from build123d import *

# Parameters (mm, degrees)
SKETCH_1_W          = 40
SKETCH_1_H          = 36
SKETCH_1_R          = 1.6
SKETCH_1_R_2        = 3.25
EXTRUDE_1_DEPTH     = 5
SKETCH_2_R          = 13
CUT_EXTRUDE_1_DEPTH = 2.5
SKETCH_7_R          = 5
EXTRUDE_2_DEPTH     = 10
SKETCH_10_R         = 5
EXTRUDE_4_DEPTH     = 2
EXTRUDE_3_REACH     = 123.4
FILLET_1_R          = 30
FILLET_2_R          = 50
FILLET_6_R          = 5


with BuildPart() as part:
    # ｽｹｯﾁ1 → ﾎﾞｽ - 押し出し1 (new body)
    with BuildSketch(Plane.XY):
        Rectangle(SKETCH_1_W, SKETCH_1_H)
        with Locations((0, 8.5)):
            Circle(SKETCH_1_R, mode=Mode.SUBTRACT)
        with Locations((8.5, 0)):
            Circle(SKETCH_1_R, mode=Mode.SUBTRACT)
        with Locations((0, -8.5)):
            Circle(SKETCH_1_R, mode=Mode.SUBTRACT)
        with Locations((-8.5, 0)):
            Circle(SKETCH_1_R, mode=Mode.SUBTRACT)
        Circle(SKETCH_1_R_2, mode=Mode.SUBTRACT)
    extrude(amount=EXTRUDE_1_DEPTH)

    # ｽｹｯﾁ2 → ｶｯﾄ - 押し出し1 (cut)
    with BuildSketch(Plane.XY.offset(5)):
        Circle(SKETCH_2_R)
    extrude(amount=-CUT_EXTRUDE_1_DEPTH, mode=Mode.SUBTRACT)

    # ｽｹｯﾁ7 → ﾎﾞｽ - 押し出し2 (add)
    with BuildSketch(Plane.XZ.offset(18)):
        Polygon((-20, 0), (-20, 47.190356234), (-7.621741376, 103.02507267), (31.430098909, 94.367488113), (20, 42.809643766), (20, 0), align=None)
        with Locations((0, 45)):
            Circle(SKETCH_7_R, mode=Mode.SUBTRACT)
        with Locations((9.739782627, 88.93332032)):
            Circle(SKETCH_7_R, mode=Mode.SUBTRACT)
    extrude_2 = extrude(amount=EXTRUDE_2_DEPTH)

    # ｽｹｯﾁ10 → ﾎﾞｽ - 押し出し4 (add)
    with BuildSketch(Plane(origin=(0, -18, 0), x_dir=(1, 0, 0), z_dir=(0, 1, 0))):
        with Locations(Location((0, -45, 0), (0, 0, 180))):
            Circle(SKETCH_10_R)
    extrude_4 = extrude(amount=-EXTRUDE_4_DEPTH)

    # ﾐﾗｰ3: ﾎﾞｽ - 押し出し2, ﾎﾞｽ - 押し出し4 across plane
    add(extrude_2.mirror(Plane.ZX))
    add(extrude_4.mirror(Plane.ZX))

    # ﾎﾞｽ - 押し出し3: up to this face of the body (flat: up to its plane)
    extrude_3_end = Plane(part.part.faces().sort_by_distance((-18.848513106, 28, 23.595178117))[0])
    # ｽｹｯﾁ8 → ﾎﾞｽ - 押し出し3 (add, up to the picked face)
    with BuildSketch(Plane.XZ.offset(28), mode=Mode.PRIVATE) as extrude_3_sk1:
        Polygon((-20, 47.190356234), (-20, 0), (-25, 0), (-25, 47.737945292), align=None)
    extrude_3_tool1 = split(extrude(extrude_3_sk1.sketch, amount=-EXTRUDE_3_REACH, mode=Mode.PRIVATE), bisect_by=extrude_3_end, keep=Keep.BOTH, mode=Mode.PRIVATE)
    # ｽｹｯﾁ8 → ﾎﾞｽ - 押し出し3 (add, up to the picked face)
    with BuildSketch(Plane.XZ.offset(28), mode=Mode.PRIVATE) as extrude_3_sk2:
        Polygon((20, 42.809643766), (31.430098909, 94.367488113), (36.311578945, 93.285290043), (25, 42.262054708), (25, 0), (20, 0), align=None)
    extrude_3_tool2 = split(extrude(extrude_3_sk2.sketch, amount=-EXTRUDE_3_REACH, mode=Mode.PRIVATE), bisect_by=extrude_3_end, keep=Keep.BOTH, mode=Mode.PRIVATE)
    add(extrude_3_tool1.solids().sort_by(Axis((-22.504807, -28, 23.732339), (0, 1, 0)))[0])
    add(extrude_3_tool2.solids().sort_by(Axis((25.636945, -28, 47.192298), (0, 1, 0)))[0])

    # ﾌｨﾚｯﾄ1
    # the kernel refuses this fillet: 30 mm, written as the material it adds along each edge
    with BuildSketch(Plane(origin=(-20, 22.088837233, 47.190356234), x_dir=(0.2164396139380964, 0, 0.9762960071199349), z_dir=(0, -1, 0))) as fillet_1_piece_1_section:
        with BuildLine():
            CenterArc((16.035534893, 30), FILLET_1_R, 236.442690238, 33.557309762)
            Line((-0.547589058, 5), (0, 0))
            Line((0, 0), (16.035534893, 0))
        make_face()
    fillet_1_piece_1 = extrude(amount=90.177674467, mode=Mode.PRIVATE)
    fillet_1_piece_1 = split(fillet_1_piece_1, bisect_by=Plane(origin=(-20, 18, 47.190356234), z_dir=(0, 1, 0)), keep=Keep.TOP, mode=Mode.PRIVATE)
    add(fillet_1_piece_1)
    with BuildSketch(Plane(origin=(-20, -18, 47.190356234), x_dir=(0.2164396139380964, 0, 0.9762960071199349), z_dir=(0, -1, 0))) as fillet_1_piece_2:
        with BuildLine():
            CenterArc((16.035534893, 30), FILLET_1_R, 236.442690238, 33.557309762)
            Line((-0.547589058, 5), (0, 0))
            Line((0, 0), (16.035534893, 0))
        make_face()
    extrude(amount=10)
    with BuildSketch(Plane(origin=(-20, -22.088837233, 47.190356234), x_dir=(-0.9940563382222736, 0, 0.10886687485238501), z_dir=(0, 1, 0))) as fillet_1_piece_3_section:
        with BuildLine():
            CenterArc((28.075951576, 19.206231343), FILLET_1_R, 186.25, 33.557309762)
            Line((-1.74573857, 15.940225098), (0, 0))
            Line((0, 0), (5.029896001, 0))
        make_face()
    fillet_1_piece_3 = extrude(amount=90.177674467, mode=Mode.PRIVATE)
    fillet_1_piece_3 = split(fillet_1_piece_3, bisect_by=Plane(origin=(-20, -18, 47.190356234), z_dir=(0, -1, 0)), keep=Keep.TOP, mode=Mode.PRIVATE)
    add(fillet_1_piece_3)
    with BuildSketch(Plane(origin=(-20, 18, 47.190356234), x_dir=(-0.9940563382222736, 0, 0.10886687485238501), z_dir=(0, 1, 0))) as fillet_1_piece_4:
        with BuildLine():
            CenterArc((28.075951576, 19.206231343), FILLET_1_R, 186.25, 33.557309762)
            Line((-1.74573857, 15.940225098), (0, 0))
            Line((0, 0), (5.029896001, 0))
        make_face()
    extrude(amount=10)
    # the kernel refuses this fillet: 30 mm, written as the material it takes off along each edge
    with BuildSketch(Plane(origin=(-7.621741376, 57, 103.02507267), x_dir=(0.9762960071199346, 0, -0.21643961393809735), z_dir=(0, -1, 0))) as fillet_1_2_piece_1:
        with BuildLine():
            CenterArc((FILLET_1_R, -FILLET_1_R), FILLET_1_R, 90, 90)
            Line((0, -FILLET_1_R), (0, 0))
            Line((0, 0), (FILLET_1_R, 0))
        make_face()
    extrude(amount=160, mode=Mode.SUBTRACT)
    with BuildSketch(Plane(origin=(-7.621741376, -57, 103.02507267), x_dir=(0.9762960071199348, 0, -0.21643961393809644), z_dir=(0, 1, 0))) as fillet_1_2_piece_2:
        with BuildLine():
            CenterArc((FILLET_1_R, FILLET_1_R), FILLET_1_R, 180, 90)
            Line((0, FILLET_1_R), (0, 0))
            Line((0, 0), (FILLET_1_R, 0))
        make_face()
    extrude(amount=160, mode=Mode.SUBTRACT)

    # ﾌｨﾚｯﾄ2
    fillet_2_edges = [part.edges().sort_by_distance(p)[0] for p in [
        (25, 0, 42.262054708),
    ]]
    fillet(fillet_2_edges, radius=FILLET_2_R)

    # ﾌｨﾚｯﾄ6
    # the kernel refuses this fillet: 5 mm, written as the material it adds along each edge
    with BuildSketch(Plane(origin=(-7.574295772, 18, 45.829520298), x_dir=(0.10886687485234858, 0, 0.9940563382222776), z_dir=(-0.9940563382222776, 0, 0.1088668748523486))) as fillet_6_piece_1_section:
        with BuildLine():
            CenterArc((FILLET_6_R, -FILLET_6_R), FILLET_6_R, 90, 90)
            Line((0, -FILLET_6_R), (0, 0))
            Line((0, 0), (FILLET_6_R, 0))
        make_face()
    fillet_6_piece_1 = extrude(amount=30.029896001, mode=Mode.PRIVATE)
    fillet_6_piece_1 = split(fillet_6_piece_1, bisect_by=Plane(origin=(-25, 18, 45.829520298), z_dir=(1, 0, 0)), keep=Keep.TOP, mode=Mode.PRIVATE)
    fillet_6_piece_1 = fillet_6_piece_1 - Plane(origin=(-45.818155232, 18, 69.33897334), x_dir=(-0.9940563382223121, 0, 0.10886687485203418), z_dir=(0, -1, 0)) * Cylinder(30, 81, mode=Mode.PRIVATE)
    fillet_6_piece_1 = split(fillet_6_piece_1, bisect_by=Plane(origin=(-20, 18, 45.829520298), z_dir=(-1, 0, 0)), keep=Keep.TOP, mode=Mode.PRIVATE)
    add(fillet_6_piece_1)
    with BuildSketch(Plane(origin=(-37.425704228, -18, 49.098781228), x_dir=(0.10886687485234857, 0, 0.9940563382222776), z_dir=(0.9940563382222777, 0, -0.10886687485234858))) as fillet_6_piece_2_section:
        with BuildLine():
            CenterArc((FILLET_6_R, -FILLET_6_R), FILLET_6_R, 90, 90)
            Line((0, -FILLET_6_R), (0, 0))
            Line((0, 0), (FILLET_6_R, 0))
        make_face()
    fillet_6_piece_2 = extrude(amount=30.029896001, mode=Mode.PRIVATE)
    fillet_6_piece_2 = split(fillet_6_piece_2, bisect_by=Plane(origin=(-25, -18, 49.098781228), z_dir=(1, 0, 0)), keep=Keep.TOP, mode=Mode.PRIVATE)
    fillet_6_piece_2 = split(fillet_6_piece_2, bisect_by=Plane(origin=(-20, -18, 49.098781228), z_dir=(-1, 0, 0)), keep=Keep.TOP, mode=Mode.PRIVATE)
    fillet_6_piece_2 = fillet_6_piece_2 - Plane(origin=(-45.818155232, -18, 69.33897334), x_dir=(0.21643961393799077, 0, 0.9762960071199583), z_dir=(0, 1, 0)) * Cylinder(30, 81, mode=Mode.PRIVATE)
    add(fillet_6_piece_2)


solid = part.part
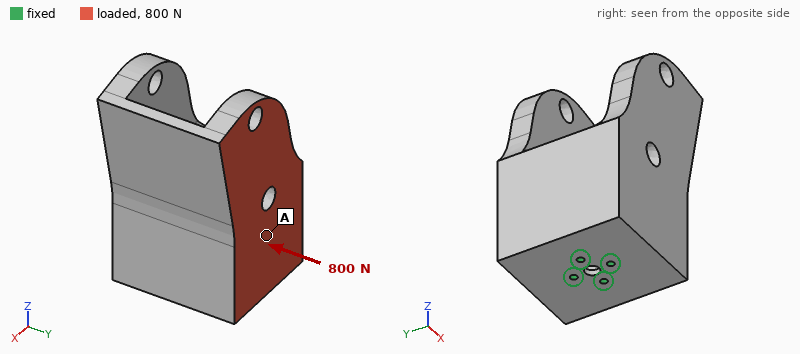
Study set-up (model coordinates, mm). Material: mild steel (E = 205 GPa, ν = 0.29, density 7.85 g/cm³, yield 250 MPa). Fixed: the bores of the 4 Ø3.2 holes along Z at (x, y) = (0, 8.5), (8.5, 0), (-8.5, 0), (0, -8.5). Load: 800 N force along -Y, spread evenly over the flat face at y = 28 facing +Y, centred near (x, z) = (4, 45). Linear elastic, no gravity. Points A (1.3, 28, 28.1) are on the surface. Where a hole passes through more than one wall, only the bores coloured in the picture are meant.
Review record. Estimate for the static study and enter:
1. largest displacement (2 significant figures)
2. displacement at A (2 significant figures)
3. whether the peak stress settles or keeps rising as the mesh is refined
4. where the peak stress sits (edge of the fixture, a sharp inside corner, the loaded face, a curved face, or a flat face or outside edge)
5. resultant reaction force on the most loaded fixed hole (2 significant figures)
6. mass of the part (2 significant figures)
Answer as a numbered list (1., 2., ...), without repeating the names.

1. 0.13 mm
2. 0.050 mm
3. keeps rising
4. edge of the fixture
5. 1.4 kN
6. 940 g
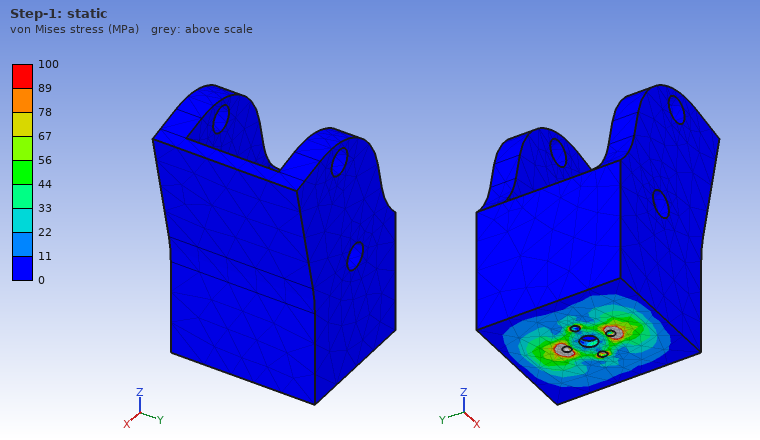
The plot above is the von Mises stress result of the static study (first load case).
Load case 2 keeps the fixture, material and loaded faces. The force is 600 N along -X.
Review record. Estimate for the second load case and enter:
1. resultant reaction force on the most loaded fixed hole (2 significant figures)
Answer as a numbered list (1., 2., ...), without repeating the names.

1. 1.1 kN
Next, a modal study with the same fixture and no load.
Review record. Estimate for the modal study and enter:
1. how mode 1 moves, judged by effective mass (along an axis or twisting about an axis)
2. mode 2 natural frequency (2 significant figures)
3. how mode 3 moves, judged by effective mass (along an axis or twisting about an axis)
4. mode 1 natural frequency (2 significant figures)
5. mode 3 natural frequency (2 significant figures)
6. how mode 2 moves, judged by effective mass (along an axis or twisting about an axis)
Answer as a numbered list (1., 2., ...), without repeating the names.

1. along X
2. 510 Hz
3. twisting about Z
4. 490 Hz
5. 2700 Hz
6. along Y
